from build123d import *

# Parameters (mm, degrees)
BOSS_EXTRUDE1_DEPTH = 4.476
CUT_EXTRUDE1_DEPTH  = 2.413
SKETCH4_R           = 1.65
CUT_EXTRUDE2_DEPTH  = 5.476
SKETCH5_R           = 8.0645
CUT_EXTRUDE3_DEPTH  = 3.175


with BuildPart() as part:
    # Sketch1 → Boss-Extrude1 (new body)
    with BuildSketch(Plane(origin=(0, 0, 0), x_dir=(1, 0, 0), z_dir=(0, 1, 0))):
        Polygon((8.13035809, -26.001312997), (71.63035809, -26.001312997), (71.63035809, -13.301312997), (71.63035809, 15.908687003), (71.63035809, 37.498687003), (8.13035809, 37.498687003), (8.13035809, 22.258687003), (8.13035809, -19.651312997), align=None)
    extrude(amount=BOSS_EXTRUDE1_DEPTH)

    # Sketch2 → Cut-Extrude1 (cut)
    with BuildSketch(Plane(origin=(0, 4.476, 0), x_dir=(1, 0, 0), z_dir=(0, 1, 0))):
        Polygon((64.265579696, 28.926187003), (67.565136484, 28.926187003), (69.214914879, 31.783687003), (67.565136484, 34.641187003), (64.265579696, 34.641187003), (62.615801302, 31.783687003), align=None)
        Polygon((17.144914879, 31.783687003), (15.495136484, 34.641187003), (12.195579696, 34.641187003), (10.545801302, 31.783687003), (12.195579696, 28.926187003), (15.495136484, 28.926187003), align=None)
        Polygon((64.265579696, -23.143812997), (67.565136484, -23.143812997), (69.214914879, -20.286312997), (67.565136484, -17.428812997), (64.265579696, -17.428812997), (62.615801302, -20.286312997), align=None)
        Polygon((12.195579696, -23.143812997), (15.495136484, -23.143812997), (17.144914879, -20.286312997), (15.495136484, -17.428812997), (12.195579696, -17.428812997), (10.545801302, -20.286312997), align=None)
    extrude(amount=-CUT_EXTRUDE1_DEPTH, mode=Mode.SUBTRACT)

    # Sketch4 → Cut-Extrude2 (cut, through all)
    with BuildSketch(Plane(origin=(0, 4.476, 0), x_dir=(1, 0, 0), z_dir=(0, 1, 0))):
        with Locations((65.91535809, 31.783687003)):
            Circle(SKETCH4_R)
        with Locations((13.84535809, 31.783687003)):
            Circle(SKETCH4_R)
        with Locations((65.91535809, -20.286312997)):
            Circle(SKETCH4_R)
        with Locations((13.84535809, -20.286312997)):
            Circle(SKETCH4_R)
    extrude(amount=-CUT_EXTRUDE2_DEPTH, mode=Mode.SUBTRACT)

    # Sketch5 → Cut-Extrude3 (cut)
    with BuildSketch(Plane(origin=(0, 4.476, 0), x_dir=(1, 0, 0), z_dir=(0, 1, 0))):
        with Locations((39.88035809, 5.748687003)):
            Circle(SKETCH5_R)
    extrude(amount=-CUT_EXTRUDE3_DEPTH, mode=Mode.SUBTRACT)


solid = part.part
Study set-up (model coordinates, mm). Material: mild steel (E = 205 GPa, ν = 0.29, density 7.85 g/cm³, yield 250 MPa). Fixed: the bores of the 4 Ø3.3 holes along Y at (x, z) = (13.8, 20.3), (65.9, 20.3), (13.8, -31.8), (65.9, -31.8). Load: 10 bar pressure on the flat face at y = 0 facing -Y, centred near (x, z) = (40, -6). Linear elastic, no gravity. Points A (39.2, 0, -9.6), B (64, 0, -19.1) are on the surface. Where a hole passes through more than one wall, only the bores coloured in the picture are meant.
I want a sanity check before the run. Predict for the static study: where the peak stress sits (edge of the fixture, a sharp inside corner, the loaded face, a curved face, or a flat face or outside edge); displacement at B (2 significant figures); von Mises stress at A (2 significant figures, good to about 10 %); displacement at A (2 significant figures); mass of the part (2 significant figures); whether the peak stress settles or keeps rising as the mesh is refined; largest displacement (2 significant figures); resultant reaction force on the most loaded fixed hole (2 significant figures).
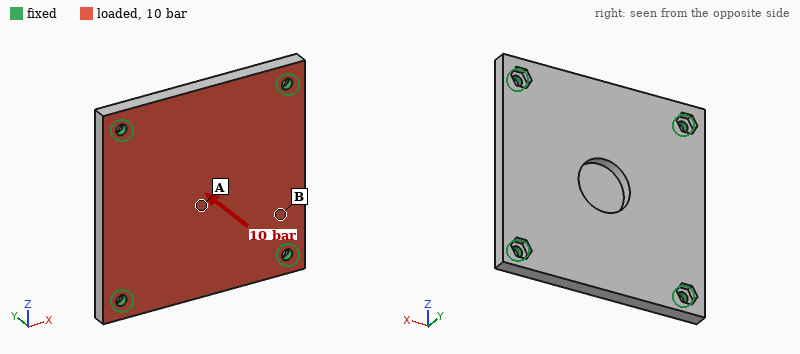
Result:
edge of the fixture
23 µm
75 MPa
61 µm
130 g
keeps rising
63 µm
1.5 kN
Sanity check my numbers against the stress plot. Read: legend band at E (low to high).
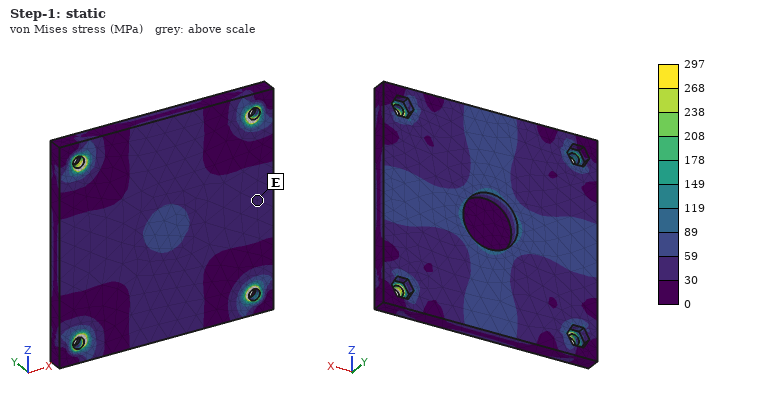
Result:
30 to 59 MPa
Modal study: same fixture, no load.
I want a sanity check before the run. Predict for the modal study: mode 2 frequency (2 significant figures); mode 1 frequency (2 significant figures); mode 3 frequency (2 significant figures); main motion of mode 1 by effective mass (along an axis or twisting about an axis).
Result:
7500 Hz
4500 Hz
7500 Hz
along Y
